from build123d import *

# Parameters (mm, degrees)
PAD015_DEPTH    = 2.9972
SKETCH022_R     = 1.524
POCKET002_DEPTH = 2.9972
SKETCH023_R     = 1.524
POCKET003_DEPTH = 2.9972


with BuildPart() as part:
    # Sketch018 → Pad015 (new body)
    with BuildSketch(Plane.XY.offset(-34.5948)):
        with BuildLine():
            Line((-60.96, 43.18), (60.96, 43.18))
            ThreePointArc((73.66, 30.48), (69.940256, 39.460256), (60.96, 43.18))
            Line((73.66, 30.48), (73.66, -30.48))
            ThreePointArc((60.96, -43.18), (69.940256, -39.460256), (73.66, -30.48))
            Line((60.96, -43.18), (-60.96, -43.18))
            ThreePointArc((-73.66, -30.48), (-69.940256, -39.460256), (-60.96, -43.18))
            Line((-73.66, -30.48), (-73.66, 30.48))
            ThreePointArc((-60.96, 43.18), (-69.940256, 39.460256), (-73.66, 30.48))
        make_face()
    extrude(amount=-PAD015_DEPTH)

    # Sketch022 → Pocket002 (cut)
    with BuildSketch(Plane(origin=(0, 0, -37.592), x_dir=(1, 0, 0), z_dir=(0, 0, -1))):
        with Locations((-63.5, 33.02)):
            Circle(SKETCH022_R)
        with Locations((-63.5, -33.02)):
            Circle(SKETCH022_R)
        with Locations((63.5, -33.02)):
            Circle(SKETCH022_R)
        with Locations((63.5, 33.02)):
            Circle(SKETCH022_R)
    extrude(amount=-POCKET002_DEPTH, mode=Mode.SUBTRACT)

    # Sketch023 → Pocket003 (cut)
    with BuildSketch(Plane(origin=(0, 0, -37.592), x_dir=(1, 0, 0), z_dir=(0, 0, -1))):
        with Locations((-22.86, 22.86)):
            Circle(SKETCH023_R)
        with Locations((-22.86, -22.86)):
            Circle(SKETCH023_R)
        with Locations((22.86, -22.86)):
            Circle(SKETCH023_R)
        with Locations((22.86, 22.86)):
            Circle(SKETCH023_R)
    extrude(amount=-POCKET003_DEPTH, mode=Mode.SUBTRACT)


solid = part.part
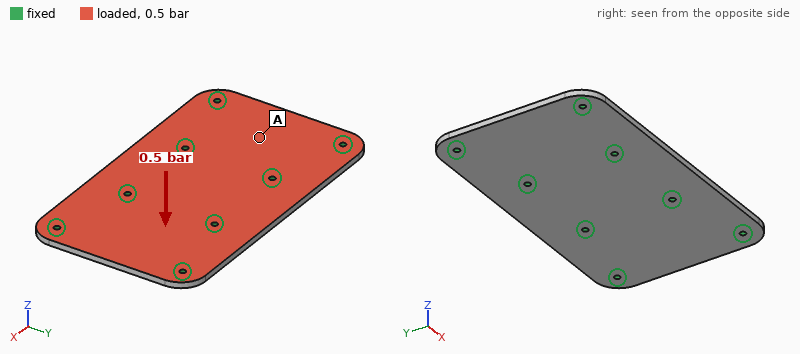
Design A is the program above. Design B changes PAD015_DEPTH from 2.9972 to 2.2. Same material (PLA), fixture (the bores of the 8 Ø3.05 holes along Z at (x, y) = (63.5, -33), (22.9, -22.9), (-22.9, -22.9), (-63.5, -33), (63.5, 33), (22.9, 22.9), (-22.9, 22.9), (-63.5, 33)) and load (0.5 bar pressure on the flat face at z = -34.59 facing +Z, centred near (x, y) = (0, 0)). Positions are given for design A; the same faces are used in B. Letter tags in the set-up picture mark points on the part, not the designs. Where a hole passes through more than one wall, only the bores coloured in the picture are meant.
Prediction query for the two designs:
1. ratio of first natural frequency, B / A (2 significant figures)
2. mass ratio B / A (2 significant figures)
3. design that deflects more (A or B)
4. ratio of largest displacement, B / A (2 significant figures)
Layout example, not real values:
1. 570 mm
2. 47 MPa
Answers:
1. 0.76
2. 0.73
3. B
4. 2.4
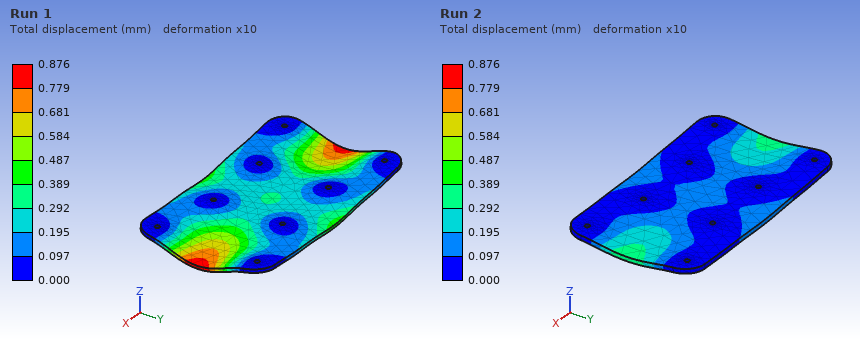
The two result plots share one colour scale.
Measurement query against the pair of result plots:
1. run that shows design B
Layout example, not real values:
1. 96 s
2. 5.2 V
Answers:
1. Run 1
